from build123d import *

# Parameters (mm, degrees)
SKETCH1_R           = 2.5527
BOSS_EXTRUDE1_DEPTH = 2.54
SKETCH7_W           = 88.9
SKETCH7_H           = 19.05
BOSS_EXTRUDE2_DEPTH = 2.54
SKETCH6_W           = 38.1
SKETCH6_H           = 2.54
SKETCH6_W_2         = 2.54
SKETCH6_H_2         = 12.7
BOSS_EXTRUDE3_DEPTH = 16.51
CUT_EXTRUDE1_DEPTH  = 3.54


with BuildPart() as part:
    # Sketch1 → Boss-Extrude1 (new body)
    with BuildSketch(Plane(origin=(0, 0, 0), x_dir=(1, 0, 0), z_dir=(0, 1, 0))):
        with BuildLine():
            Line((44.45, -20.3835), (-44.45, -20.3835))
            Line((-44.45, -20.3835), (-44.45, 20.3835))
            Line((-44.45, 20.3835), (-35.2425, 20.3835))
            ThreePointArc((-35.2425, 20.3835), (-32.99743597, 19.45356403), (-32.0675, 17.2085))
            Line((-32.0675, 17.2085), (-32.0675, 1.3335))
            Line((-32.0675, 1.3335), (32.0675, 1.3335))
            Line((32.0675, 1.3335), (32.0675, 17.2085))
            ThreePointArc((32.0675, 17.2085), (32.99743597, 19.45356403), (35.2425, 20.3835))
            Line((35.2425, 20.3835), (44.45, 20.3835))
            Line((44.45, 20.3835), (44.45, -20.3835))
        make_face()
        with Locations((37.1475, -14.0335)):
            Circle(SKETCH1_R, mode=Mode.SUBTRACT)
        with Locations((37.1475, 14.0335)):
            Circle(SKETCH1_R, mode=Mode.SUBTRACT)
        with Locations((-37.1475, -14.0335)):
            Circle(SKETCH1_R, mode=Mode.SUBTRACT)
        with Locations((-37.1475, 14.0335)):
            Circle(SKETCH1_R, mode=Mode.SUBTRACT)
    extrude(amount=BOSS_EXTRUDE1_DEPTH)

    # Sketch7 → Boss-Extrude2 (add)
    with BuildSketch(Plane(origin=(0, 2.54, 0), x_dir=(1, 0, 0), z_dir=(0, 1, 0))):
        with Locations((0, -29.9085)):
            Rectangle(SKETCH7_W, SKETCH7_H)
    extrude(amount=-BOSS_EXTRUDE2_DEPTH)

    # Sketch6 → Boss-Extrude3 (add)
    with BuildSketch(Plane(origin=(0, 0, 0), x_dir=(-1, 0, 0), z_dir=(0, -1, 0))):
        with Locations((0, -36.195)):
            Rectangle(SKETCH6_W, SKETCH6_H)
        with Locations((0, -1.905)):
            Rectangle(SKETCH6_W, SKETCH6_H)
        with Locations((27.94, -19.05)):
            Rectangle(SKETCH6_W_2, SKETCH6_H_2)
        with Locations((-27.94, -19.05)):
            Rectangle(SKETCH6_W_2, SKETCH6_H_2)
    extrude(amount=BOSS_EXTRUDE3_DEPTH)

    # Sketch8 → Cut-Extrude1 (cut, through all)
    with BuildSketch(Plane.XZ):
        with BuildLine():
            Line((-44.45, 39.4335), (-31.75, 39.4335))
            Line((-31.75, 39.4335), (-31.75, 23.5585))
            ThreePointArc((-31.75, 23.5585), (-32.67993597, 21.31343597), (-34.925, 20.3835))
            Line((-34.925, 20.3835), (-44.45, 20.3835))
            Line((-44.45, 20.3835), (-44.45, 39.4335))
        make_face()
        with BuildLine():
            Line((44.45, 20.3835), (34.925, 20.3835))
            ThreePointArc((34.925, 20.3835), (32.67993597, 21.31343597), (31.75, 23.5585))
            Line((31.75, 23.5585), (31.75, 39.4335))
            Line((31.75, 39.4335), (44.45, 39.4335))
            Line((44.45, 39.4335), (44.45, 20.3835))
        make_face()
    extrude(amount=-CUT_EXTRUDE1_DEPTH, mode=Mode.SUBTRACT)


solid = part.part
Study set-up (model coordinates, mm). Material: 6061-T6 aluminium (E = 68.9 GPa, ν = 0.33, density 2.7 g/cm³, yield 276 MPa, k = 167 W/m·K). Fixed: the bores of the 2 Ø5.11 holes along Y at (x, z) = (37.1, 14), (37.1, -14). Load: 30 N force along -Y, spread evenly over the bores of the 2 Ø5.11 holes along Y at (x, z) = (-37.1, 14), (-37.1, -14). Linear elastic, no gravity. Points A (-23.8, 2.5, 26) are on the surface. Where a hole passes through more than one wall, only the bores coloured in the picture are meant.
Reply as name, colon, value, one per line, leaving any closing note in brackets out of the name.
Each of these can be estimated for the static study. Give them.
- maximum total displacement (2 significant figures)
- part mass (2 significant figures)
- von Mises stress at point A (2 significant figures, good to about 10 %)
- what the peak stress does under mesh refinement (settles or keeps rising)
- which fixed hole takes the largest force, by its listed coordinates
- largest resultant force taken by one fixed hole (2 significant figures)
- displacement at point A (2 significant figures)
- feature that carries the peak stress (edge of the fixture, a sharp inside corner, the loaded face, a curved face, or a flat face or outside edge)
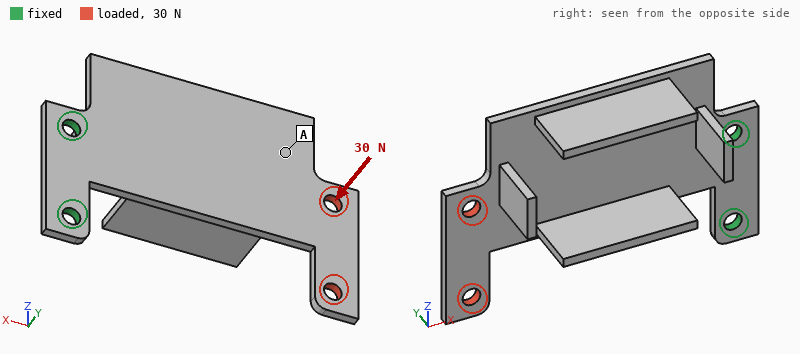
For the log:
maximum total displacement: 1.3 mm
part mass: 36 g
von Mises stress at point A: 9.9 MPa
what the peak stress does under mesh refinement: keeps rising
which fixed hole takes the largest force, by its listed coordinates: (37.1, 14)
largest resultant force taken by one fixed hole: 38 N
displacement at point A: 0.69 mm
feature that carries the peak stress: edge of the fixture
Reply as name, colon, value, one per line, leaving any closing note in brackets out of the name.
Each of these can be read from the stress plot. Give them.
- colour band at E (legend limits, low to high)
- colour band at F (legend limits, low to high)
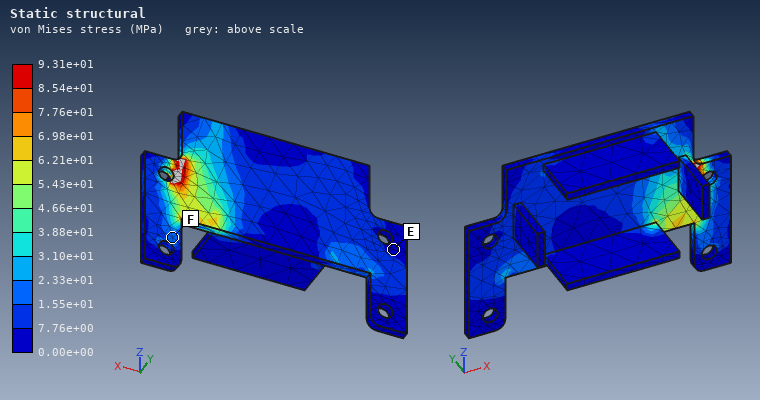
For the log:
colour band at E: 0.00e+00 to 7.76e+00 MPa
colour band at F: 1.55e+01 to 2.33e+01 MPa
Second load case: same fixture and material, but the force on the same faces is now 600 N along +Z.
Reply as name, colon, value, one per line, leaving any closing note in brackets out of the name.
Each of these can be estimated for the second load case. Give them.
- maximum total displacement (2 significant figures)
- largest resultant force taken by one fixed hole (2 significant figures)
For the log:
maximum total displacement: 0.54 mm
largest resultant force taken by one fixed hole: 1.4 kN
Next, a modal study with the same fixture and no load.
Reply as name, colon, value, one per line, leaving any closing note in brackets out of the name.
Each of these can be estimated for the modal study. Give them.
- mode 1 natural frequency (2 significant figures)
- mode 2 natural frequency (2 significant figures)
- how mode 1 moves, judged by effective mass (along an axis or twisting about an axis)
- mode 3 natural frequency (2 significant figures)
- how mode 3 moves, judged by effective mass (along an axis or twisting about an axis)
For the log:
mode 1 natural frequency: 270 Hz
mode 2 natural frequency: 740 Hz
how mode 1 moves, judged by effective mass: along Y
mode 3 natural frequency: 1600 Hz
how mode 3 moves, judged by effective mass: along Z
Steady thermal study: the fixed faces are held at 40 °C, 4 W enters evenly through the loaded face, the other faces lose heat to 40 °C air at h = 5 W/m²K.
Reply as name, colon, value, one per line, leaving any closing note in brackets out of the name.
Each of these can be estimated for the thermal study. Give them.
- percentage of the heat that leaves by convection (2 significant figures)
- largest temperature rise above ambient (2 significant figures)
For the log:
percentage of the heat that leaves by convection: 13 %
largest temperature rise above ambient: 26 K
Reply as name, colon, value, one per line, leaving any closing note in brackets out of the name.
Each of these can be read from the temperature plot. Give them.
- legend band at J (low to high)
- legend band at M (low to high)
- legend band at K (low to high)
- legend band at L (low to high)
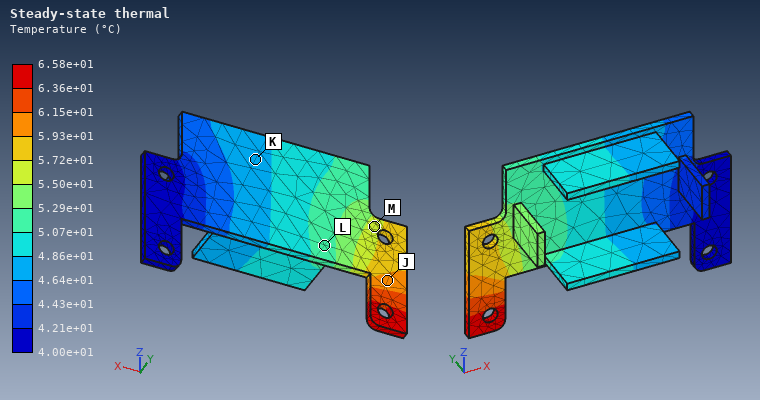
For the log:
legend band at J: 5.93e+01 to 6.15e+01 °C
legend band at M: 5.50e+01 to 5.72e+01 °C
legend band at K: 4.64e+01 to 4.86e+01 °C
legend band at L: 5.07e+01 to 5.29e+01 °C
